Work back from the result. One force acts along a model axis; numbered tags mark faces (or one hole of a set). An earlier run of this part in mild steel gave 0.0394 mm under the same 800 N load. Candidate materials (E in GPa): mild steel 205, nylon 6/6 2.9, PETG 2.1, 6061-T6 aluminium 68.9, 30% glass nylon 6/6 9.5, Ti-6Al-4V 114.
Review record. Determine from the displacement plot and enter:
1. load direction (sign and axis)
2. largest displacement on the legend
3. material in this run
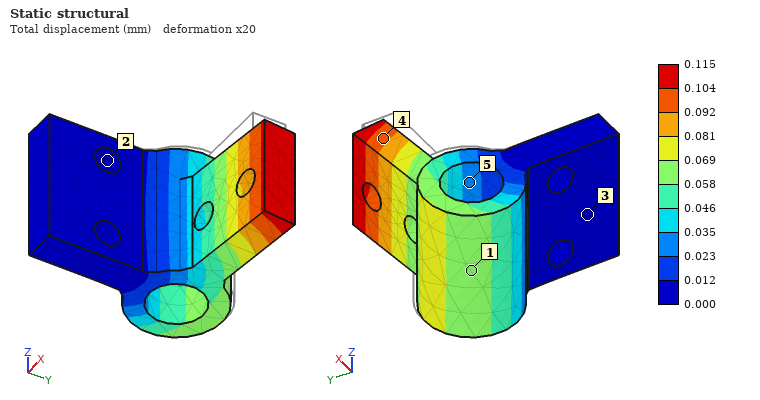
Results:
-X
0.115 mm
6061-T6 aluminium
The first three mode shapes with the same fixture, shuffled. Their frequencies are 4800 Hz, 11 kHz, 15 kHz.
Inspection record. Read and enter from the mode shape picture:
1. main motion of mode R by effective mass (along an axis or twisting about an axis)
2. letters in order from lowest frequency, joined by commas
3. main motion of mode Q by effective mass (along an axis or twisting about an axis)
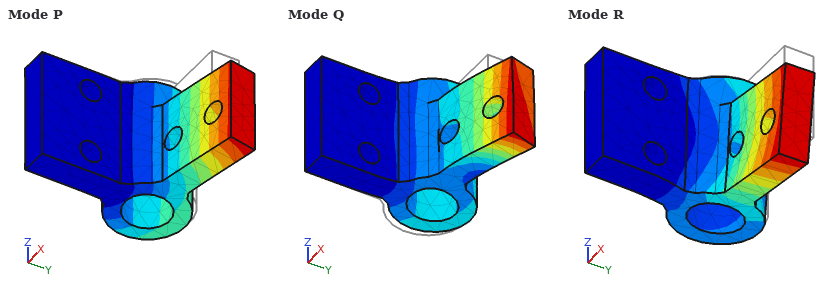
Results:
along Z
P, R, Q
along X
